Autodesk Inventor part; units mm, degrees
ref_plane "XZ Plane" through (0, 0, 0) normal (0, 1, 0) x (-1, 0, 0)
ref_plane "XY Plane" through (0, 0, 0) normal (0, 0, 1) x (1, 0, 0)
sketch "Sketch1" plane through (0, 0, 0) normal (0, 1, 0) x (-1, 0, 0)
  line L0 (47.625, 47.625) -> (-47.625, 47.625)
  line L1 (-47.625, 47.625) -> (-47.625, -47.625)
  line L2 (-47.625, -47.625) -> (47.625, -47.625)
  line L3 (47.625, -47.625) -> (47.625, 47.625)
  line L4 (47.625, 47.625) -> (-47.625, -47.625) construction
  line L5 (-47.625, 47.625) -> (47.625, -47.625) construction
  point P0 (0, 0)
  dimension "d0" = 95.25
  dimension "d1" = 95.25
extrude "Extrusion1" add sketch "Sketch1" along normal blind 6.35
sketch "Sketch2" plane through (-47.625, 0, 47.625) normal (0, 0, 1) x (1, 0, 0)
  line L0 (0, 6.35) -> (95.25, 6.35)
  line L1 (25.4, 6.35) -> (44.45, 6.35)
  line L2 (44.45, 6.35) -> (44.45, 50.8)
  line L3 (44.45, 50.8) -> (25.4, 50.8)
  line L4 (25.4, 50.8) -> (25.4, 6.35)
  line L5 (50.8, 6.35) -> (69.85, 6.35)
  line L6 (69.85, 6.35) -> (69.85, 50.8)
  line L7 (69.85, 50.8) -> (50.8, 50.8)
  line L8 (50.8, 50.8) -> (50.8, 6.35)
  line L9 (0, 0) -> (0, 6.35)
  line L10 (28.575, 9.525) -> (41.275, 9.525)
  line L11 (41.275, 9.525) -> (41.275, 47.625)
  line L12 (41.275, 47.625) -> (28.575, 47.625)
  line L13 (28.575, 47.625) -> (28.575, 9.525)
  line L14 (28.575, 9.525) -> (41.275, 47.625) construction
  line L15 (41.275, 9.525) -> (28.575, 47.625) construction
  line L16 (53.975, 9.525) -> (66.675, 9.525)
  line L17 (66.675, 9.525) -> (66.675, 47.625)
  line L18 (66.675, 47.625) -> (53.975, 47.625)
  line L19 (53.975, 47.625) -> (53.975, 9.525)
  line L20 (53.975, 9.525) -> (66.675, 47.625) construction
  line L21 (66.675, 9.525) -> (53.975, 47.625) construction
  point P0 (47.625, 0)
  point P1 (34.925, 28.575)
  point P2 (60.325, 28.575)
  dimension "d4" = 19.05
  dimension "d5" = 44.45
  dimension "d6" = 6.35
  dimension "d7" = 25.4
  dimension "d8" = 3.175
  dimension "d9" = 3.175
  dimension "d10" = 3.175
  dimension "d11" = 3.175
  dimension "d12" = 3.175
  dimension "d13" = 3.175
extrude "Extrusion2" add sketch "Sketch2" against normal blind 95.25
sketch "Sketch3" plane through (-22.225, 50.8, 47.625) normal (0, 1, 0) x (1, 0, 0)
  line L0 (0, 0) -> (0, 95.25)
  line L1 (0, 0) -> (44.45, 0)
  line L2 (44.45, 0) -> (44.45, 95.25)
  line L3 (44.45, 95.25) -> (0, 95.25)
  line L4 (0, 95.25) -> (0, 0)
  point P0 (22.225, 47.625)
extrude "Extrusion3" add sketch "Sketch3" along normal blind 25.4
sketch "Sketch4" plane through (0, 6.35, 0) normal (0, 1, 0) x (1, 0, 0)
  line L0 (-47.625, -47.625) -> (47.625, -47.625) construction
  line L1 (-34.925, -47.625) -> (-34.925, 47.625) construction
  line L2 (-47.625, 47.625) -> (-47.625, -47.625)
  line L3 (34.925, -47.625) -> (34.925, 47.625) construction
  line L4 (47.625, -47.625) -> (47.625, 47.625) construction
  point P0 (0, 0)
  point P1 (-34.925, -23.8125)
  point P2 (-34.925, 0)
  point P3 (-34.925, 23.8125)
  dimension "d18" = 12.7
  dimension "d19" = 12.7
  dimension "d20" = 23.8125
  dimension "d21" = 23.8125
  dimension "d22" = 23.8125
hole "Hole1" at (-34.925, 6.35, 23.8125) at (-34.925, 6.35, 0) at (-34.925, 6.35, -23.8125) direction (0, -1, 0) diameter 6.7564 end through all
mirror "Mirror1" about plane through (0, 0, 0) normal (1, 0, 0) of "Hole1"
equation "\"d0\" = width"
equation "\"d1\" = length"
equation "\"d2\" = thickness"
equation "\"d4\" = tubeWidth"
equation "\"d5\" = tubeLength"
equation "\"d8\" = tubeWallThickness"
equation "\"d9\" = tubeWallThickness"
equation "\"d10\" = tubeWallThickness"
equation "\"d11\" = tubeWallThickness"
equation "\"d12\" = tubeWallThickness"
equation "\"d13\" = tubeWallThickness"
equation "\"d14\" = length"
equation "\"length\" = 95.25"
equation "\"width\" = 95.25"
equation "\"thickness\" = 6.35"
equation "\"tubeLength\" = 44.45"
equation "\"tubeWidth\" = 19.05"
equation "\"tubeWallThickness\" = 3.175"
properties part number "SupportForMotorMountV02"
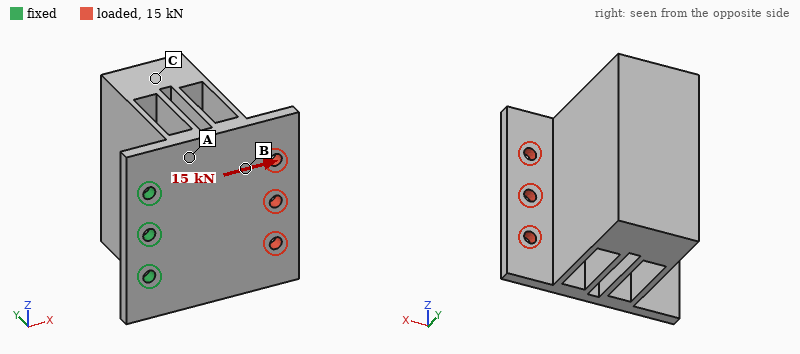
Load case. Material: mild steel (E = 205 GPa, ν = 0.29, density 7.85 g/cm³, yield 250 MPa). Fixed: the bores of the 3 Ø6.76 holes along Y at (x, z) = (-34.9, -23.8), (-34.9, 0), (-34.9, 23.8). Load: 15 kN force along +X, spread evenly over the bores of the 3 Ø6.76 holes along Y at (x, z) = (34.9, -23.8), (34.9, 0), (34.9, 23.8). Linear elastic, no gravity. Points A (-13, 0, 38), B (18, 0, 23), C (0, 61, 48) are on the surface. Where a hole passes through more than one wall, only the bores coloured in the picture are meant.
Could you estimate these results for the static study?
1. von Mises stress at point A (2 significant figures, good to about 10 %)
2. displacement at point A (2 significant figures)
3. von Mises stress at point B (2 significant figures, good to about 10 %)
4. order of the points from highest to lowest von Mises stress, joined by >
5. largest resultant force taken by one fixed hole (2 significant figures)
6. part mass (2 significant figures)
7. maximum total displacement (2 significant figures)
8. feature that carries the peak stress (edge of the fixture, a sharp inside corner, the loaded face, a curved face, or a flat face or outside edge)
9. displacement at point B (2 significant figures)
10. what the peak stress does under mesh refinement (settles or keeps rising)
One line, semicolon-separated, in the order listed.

20 MPa; 4.7 µm; 35 MPa; B > A > C; 5.4 kN; 1.8 kg; 20 µm; edge of the fixture; 10 µm; keeps rising
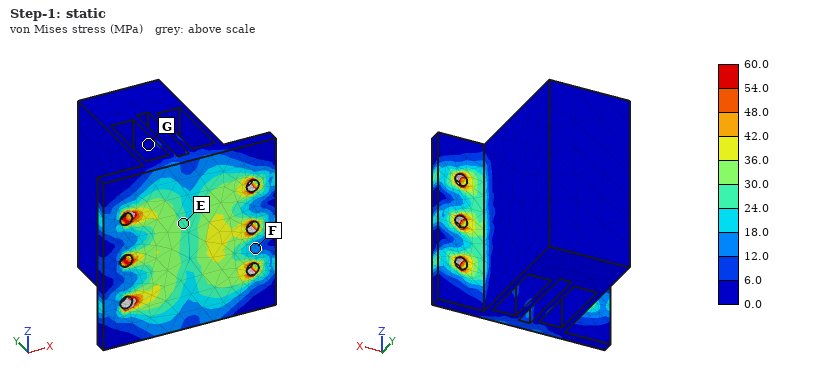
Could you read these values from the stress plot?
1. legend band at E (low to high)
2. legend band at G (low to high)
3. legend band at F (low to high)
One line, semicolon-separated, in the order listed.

24.0 to 30.0 MPa; 0.0 to 6.0 MPa; 12.0 to 18.0 MPa
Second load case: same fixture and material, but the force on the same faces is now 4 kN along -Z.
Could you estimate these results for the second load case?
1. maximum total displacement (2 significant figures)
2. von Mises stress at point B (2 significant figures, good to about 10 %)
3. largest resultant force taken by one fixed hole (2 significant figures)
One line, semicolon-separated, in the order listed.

22 µm; 11 MPa; 5.4 kN
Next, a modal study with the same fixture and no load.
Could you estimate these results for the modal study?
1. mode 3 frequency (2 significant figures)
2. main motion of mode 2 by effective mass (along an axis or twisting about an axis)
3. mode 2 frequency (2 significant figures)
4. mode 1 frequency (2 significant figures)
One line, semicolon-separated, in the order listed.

1600 Hz; along Z; 1100 Hz; 320 Hz
